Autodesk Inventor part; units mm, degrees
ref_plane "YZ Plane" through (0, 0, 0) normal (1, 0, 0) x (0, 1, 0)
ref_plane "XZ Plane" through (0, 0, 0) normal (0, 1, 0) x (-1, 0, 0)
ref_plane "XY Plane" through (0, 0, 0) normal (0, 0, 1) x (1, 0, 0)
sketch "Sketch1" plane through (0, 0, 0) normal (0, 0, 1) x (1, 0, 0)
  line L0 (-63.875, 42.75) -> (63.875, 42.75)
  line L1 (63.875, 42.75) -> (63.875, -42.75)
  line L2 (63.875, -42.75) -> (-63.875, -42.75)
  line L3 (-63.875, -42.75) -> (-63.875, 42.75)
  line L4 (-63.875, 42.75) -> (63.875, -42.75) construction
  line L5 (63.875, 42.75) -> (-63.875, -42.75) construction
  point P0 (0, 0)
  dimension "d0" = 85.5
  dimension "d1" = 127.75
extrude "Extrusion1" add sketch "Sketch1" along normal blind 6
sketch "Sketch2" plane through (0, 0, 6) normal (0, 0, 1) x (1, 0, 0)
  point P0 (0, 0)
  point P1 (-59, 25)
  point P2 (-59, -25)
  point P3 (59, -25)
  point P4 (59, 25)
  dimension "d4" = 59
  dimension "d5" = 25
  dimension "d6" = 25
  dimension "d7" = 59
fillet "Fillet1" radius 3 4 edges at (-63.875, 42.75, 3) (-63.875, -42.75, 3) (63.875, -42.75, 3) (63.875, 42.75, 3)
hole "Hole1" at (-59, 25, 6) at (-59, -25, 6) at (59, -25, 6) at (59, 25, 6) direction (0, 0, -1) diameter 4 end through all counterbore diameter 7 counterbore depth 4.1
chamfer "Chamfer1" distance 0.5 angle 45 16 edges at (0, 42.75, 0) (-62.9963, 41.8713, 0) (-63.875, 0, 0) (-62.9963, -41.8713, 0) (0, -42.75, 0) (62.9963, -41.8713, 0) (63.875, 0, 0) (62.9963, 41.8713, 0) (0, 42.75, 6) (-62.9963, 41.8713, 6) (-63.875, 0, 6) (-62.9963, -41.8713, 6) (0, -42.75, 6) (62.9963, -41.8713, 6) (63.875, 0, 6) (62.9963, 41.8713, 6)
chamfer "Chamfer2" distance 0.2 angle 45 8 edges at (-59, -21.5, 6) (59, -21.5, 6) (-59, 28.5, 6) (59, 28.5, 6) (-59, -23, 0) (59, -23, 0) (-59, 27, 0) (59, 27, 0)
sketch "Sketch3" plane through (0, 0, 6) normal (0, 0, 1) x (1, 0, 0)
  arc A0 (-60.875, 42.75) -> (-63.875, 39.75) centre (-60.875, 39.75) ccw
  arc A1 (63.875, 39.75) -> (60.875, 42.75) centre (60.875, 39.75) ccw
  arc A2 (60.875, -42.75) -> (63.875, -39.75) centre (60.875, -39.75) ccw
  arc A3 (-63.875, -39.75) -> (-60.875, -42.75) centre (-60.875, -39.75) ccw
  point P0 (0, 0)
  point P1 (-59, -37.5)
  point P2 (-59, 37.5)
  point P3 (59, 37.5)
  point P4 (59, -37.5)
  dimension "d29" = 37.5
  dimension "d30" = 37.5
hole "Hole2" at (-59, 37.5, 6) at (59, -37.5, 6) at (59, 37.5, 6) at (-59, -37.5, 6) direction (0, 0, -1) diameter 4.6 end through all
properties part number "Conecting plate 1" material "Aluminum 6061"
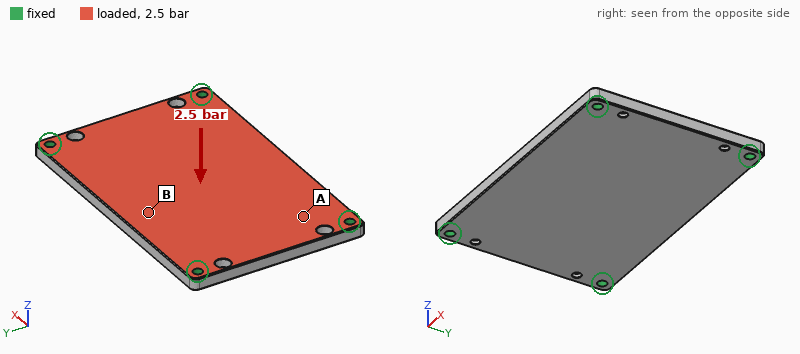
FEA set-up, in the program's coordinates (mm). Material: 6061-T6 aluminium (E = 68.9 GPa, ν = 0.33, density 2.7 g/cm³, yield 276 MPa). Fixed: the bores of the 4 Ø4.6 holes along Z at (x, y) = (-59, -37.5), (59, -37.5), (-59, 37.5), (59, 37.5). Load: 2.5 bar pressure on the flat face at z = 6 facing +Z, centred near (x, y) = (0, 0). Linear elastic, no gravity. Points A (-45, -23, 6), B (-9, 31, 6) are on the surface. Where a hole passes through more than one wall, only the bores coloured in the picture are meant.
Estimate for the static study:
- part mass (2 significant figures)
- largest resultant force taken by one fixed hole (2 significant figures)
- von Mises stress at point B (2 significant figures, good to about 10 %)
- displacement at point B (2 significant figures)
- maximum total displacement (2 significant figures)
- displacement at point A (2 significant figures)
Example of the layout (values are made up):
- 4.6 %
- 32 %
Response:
- 170 g
- 660 N
- 30 MPa
- 0.16 mm
- 0.18 mm
- 0.057 mm
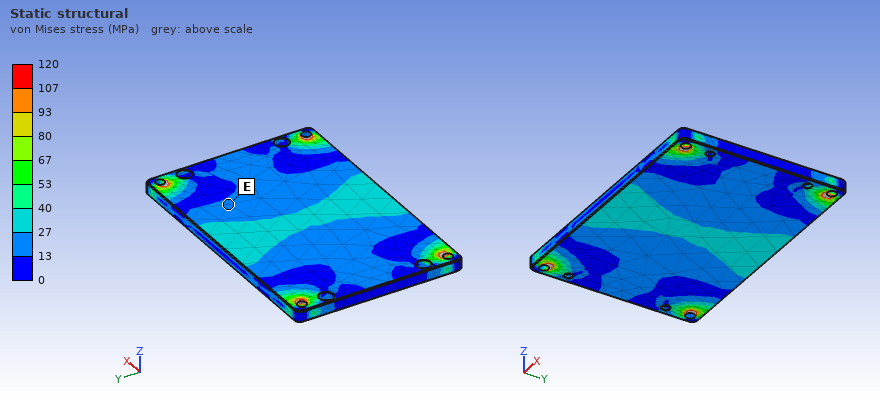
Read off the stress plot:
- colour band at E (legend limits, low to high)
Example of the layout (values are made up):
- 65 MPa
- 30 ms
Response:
- 13 to 27 MPa
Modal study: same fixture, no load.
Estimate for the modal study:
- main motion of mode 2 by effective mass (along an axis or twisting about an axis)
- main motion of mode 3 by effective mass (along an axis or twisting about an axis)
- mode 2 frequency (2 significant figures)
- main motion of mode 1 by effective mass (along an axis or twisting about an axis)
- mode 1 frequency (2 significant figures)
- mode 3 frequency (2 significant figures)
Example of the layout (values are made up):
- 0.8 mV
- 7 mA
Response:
- twisting about X
- twisting about Y
- 2900 Hz
- along Z
- 1700 Hz
- 4300 Hz
